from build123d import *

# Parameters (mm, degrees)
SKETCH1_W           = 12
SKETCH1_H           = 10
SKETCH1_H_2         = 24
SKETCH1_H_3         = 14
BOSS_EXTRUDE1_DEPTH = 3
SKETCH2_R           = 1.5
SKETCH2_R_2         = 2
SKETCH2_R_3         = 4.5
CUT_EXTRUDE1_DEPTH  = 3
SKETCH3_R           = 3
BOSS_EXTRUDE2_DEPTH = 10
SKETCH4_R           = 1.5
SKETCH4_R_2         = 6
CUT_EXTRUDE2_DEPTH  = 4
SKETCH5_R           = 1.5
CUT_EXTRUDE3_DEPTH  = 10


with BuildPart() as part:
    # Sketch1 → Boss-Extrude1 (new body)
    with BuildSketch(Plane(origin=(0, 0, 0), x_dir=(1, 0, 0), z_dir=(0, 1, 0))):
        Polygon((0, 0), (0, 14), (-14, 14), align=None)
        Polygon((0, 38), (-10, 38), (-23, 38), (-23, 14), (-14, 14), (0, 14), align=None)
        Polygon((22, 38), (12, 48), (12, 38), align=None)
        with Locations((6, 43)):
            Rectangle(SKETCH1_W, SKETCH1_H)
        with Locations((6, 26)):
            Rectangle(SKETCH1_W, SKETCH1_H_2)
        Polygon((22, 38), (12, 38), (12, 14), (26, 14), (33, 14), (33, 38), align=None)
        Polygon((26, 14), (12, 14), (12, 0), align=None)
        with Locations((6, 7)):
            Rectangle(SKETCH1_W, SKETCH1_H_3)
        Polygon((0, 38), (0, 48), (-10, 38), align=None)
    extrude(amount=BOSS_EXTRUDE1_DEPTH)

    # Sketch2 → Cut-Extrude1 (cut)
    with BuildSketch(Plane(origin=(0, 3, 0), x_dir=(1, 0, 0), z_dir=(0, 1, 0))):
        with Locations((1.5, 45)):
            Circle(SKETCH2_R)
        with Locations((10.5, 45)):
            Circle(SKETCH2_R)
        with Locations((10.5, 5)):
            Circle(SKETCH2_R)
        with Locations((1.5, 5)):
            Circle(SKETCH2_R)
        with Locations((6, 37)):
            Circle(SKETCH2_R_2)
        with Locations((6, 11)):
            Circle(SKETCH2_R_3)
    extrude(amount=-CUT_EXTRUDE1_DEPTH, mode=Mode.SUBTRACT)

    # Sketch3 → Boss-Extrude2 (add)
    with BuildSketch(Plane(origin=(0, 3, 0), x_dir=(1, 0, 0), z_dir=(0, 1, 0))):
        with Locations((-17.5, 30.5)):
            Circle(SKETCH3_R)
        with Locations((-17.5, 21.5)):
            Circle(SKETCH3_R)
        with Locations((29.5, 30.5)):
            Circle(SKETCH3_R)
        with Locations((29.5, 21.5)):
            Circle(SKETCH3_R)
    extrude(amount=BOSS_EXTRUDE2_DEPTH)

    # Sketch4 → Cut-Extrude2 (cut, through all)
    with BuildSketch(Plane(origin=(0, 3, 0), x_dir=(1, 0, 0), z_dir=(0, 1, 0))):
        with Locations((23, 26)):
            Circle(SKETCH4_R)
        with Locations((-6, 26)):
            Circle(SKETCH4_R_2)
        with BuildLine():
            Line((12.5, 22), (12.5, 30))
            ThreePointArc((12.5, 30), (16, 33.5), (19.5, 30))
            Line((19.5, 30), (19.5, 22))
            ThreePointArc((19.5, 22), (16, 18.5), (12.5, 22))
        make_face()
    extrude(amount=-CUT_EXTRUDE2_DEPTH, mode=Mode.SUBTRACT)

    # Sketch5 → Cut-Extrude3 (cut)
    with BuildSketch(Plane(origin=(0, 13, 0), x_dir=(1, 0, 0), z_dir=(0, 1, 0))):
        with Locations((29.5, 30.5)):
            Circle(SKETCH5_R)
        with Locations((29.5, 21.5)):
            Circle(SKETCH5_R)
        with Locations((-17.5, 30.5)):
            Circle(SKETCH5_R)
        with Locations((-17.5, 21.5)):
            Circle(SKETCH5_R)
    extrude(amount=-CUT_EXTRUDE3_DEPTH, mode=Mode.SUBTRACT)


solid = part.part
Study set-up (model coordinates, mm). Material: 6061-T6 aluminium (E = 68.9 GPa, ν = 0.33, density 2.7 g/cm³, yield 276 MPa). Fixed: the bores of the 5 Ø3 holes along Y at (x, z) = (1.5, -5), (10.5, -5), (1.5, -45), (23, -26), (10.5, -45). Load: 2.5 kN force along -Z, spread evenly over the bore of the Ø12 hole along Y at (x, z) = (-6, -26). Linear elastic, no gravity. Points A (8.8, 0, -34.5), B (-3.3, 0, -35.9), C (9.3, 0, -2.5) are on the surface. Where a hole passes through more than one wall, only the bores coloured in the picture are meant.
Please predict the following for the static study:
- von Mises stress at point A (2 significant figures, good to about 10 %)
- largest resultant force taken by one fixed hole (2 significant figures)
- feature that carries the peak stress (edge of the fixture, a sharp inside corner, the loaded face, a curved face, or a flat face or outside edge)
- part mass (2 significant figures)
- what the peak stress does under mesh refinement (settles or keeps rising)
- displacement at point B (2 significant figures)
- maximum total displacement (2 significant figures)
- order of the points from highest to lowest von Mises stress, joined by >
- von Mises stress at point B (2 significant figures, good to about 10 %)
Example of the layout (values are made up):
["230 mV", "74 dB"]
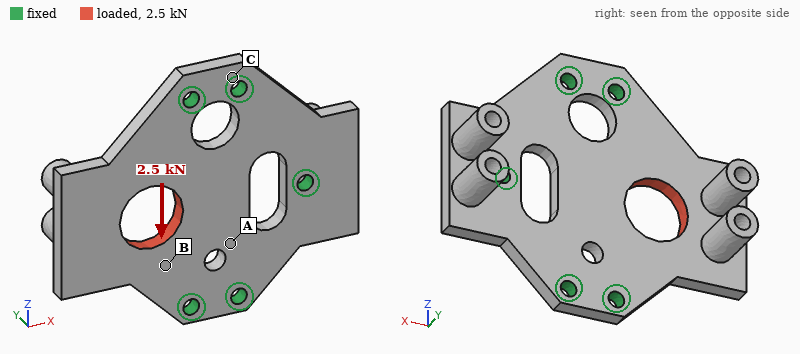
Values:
["20 MPa", "1.1 kN", "edge of the fixture", "15 g", "keeps rising", "7.4 µm", "19 µm", "B > A > C", "36 MPa"]
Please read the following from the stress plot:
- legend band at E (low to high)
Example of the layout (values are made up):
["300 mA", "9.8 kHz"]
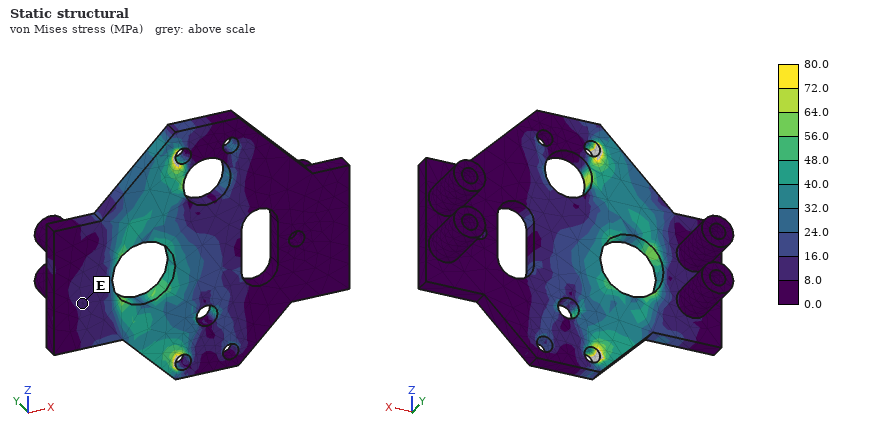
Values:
["8.0 to 16.0 MPa"]
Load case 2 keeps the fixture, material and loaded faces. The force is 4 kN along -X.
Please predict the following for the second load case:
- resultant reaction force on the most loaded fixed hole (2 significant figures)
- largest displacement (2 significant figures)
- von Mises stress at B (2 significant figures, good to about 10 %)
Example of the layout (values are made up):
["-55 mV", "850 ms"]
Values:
["1.1 kN", "26 µm", "44 MPa"]
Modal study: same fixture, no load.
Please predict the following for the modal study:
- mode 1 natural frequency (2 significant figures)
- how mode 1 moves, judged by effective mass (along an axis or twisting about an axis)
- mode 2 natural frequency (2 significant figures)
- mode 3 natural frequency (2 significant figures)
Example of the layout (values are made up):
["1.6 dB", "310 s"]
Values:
["2600 Hz", "along Y", "7700 Hz", "9600 Hz"]
